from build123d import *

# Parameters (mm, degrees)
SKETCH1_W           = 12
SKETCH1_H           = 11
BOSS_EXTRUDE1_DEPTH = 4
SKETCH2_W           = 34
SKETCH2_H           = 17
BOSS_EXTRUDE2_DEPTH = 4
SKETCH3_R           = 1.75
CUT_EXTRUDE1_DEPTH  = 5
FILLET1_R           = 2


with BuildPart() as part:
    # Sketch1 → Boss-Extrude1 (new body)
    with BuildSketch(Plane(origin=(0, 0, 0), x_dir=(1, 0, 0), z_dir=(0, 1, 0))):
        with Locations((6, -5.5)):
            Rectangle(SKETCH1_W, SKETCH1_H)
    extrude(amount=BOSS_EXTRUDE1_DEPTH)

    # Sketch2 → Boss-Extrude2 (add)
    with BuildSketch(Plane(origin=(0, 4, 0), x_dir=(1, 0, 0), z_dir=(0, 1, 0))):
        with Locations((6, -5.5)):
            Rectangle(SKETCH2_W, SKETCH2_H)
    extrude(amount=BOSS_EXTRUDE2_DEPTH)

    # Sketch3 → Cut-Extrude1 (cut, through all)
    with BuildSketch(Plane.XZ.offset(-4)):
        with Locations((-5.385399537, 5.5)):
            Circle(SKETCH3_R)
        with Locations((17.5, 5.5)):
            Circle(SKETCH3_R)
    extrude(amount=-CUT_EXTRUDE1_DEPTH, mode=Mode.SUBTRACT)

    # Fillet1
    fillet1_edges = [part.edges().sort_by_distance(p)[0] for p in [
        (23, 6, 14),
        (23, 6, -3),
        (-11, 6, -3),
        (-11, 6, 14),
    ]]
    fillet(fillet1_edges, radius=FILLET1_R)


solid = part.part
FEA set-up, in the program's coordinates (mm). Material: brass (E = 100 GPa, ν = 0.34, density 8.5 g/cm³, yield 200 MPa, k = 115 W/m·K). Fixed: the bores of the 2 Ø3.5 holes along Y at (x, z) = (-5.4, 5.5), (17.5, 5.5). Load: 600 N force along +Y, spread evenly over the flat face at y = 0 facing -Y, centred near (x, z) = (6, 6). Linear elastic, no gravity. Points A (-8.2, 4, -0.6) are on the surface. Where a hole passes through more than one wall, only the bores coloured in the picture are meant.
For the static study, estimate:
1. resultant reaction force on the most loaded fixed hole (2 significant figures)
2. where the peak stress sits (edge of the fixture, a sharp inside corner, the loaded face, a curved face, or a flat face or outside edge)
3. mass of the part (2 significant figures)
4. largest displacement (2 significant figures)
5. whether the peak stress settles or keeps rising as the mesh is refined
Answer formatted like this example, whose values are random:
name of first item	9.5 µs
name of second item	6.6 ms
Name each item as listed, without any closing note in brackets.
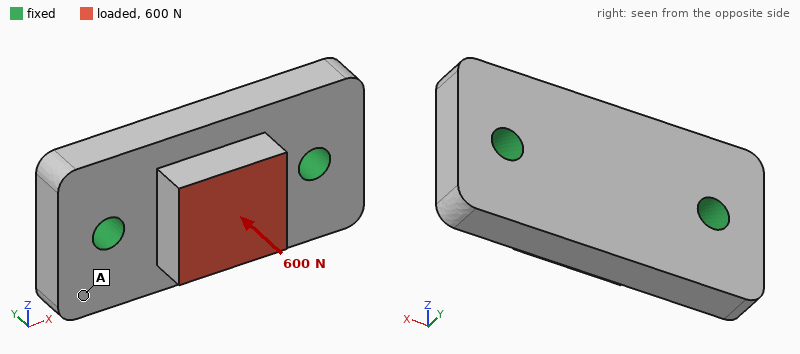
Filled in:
resultant reaction force on the most loaded fixed hole	320 N
where the peak stress sits	edge of the fixture
mass of the part	23 g
largest displacement	3.0 µm
whether the peak stress settles or keeps rising as the mesh is refined	keeps rising
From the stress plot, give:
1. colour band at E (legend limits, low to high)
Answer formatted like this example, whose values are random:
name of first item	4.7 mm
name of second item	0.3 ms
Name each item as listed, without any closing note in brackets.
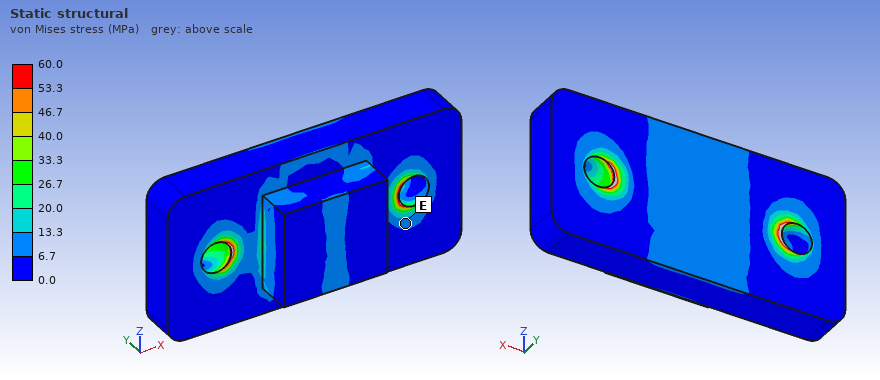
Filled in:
colour band at E	6.7 to 13.3 MPa
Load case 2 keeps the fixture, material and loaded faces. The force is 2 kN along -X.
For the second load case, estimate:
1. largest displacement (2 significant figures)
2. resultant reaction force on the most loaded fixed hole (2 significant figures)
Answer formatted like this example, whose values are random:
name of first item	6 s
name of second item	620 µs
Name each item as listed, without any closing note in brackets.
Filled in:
largest displacement	8.6 µm
resultant reaction force on the most loaded fixed hole	1.2 kN
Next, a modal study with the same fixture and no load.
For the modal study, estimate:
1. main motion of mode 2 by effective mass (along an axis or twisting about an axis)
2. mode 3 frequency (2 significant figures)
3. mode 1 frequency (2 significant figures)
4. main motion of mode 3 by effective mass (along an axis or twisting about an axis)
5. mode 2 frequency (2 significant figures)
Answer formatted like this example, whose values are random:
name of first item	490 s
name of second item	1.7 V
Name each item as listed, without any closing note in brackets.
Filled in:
main motion of mode 2 by effective mass	along Y
mode 3 frequency	30 kHz
mode 1 frequency	16 kHz
main motion of mode 3 by effective mass	along Z
mode 2 frequency	21 kHz
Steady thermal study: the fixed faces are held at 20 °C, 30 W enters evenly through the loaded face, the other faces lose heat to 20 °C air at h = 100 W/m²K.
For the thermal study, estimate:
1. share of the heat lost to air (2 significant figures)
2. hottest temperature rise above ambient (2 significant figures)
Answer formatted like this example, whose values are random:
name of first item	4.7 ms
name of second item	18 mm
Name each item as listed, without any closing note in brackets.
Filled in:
share of the heat lost to air	4.6 %
hottest temperature rise above ambient	25 K
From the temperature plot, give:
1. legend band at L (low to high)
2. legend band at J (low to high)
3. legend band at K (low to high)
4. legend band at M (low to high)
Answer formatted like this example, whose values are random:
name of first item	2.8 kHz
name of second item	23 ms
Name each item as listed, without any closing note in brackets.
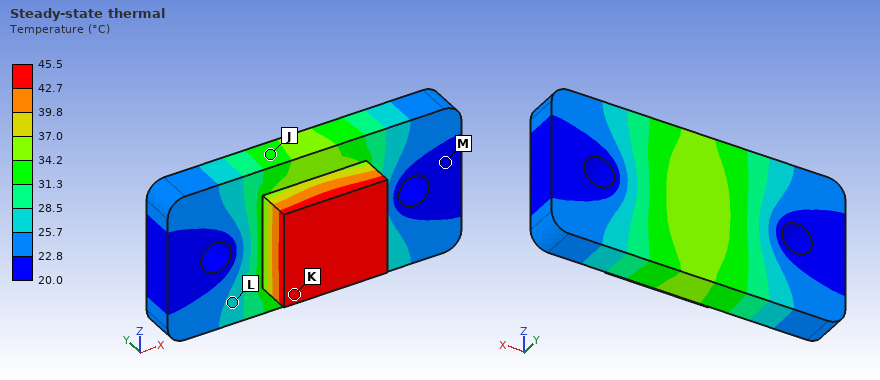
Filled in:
legend band at L	25.7 to 28.5 °C
legend band at J	31.3 to 34.2 °C
legend band at K	42.7 to 45.5 °C
legend band at M	20.0 to 22.8 °C
